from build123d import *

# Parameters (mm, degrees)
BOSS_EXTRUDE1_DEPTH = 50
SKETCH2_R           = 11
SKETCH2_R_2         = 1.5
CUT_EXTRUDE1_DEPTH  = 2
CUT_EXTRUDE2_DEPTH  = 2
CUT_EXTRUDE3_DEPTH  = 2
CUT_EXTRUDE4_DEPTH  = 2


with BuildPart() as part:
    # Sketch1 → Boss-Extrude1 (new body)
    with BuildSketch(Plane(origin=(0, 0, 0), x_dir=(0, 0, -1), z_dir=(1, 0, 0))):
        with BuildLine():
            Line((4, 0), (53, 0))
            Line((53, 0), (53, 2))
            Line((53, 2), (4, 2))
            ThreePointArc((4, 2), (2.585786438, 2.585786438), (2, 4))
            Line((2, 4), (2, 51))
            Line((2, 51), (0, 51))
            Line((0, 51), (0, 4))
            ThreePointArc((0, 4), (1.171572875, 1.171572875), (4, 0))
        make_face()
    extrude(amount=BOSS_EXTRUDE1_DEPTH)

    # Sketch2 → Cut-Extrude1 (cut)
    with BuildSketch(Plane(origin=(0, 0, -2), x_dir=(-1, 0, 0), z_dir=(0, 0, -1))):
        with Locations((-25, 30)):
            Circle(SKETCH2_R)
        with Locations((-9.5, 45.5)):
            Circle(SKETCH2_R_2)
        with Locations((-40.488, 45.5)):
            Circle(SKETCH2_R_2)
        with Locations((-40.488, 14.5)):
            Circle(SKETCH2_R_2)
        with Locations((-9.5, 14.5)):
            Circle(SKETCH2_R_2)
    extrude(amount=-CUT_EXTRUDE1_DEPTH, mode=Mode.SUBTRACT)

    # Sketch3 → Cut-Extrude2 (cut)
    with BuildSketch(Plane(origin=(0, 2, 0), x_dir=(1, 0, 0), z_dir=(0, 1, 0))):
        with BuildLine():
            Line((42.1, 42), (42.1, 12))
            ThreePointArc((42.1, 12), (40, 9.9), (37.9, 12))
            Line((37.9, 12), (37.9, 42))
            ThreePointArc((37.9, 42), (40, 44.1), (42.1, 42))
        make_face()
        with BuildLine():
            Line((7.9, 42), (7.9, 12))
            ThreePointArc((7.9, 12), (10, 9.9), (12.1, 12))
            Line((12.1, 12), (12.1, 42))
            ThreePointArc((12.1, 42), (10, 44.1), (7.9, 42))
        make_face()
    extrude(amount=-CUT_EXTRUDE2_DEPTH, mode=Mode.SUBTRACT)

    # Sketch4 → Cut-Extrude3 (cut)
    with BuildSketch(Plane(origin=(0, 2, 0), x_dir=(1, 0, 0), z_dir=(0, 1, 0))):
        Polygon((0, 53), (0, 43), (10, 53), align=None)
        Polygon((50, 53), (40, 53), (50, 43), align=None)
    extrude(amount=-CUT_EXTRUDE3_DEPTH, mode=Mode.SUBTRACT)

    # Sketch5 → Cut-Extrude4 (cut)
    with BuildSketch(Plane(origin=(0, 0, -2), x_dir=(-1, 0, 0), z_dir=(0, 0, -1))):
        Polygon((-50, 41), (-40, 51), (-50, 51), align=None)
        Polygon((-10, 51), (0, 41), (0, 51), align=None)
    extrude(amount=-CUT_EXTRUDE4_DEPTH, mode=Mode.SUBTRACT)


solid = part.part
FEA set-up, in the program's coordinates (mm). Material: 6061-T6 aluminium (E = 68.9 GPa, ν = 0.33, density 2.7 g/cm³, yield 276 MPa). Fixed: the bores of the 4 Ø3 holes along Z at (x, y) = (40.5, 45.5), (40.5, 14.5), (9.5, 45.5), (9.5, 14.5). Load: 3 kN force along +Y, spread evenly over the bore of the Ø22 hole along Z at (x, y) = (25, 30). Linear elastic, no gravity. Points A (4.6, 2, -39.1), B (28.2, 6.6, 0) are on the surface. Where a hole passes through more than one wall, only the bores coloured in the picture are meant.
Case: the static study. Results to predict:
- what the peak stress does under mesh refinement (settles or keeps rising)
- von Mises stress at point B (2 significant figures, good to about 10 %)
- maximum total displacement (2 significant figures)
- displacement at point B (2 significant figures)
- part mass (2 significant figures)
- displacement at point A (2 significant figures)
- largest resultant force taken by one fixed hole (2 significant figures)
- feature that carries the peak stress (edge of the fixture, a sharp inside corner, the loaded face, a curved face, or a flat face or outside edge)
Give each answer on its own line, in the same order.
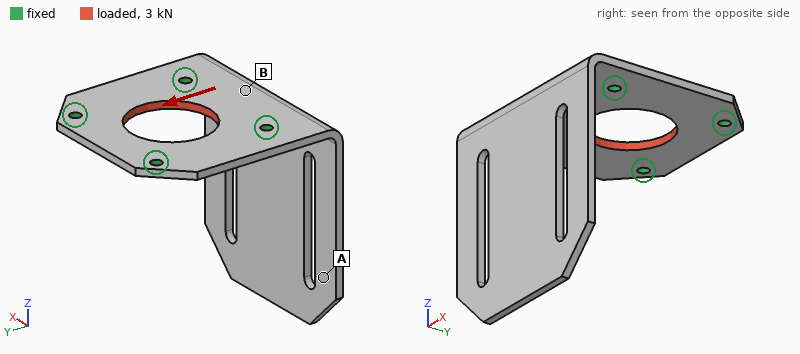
keeps rising
11 MPa
15 µm
5.7 µm
22 g
4.6 µm
790 N
edge of the fixture
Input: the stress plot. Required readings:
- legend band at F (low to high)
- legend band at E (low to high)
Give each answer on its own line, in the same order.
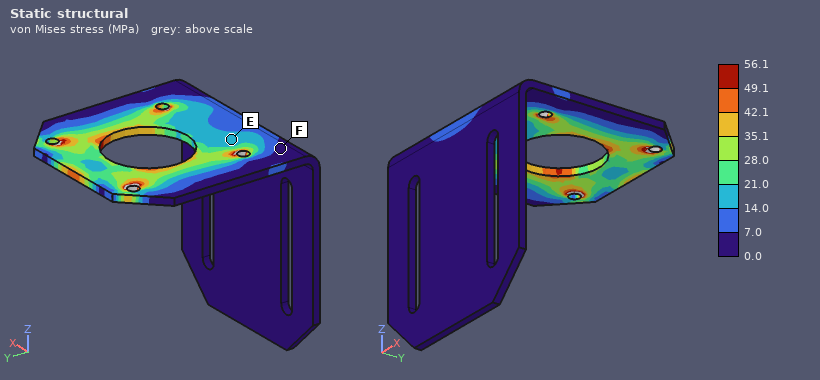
0.0 to 7.0 MPa
14.0 to 21.0 MPa
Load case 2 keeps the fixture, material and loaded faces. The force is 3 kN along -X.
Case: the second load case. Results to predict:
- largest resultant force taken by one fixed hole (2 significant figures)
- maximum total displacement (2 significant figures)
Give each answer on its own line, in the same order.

780 N
11 µm
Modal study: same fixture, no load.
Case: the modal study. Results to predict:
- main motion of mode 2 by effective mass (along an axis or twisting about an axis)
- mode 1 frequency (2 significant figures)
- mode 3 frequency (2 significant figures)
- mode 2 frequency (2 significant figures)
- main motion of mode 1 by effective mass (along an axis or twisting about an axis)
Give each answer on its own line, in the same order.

along X
470 Hz
1900 Hz
1300 Hz
along Y
